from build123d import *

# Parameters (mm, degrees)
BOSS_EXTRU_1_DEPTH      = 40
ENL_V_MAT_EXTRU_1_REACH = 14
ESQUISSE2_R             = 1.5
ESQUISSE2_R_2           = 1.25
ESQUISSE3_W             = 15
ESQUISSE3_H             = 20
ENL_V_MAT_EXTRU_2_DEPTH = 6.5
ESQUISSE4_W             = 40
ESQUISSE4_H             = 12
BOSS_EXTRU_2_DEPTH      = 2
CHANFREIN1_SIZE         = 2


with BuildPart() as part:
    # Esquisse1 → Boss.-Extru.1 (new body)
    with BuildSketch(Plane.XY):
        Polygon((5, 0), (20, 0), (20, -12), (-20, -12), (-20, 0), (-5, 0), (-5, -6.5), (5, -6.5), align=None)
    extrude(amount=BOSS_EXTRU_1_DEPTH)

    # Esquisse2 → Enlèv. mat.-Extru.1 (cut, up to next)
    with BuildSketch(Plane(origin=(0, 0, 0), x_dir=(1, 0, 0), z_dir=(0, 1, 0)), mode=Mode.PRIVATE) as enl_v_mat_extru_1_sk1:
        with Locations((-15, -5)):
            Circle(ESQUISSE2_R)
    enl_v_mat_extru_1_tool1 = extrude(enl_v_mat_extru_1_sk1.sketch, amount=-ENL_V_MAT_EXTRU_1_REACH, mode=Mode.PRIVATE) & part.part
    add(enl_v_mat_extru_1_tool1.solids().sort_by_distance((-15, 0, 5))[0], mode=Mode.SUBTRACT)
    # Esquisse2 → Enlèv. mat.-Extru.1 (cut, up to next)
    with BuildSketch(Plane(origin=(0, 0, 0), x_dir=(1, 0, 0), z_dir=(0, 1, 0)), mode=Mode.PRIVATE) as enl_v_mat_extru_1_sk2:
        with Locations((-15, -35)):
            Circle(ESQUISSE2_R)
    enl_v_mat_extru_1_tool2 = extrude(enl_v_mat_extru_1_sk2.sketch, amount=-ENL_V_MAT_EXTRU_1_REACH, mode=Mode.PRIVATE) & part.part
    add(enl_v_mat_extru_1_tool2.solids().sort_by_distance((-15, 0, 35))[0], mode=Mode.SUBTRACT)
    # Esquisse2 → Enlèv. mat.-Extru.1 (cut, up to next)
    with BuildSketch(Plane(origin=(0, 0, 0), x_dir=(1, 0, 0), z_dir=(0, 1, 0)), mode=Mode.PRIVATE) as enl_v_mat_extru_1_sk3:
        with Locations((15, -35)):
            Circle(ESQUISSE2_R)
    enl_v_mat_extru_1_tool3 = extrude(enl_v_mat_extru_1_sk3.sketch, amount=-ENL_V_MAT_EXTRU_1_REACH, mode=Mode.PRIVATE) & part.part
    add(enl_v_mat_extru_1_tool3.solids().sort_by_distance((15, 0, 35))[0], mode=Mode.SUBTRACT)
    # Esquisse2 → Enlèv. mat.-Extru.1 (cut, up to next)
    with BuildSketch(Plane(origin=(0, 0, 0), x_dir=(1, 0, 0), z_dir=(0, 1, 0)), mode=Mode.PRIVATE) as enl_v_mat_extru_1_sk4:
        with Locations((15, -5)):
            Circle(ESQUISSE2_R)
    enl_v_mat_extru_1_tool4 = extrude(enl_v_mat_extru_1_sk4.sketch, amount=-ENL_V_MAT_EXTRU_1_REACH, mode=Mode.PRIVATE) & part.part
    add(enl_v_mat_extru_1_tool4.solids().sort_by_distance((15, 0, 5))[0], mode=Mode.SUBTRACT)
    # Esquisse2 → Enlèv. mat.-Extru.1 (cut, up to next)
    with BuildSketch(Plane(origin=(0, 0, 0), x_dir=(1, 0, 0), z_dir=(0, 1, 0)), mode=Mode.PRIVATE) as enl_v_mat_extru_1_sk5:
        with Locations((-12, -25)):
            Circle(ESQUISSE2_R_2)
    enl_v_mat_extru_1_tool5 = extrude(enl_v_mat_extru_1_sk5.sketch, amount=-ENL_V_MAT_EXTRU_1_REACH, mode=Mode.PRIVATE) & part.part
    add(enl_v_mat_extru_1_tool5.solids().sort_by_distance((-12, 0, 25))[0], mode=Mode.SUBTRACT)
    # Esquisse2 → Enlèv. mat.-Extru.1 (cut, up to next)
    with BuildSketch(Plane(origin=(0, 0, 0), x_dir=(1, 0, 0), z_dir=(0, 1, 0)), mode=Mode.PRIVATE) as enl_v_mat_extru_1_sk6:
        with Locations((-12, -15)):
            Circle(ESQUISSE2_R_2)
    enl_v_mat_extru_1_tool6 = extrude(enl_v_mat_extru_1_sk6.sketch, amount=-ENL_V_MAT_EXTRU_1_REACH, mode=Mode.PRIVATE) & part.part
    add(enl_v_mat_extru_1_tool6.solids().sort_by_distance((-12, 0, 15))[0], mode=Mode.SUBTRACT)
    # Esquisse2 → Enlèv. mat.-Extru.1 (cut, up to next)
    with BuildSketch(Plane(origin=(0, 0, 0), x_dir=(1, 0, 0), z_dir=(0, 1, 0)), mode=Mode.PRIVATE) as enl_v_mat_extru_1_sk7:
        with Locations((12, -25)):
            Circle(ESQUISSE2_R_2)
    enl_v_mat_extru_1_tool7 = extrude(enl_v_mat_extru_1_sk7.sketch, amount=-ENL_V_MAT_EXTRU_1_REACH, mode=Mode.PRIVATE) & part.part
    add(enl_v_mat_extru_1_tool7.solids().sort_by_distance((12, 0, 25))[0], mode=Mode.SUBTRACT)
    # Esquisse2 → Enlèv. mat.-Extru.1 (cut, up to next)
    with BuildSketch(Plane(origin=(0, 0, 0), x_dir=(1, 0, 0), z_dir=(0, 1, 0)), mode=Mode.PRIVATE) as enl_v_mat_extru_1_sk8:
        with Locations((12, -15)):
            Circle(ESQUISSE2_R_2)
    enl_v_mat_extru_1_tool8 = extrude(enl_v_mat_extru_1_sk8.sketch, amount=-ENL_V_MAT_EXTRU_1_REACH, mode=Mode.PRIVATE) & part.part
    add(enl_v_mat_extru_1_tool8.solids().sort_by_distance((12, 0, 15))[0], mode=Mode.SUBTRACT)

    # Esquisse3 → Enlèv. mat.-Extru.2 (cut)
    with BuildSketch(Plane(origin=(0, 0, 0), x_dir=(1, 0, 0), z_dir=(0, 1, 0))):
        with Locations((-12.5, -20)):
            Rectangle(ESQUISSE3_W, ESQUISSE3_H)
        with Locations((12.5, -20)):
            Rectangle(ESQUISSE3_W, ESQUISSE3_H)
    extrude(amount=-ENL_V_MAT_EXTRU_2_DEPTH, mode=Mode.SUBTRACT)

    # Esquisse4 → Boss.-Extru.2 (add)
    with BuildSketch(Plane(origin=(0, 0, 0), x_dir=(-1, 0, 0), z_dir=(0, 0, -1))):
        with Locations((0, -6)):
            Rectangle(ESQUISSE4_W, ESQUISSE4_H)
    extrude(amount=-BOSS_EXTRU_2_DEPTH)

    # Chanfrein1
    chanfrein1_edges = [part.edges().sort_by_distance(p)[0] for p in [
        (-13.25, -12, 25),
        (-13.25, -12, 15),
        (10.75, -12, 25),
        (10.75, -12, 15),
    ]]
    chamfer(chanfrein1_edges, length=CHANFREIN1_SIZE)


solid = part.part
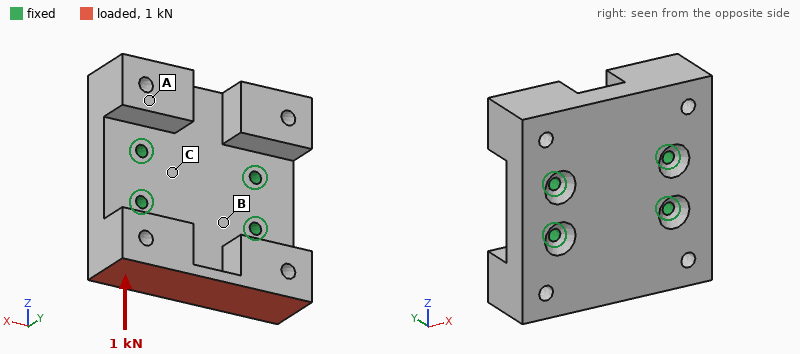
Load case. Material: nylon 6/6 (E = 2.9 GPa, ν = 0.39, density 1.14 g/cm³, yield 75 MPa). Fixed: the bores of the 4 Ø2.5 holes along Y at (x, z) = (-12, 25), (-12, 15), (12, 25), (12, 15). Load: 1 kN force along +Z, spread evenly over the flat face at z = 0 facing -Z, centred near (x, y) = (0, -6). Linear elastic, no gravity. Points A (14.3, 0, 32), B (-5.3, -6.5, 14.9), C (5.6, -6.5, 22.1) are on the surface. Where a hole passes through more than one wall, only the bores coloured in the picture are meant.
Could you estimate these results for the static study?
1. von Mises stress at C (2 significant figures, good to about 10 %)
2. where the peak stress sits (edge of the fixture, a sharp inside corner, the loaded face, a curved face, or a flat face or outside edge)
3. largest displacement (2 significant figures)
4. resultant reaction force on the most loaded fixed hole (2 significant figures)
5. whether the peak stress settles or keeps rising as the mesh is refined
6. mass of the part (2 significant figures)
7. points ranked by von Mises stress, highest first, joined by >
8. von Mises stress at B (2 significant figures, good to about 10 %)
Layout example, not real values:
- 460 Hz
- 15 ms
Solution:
- 4.7 MPa
- edge of the fixture
- 0.38 mm
- 410 N
- keeps rising
- 14 g
- B > C > A
- 12 MPa
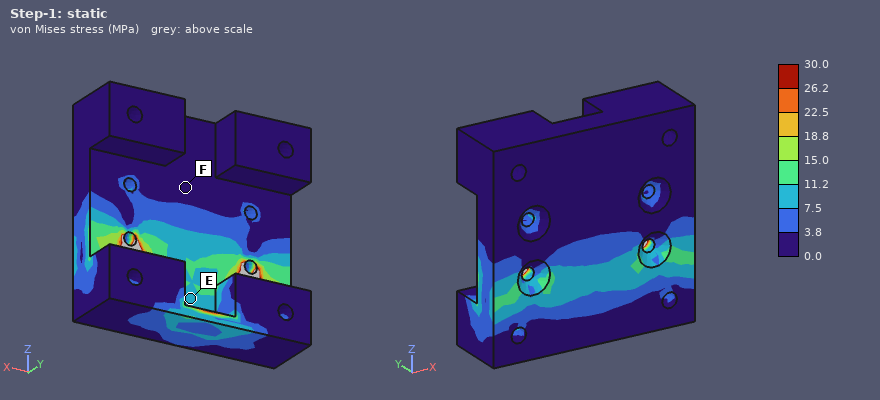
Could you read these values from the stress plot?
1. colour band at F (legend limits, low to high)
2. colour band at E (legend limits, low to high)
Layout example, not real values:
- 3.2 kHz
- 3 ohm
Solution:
- 0.0 to 3.8 MPa
- 7.5 to 11.2 MPa
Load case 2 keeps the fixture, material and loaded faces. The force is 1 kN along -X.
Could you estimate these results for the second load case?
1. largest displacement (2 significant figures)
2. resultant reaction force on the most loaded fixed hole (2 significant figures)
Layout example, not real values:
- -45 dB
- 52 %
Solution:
- 0.20 mm
- 650 N
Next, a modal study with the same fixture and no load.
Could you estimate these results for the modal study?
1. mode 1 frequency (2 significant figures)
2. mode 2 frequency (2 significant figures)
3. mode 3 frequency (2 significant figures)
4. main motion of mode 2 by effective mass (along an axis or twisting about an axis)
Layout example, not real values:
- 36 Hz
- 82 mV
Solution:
- 2800 Hz
- 3000 Hz
- 4100 Hz
- along Y
